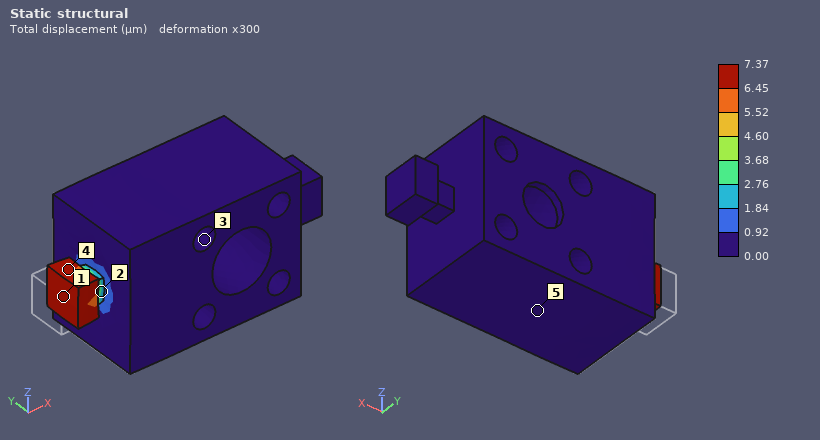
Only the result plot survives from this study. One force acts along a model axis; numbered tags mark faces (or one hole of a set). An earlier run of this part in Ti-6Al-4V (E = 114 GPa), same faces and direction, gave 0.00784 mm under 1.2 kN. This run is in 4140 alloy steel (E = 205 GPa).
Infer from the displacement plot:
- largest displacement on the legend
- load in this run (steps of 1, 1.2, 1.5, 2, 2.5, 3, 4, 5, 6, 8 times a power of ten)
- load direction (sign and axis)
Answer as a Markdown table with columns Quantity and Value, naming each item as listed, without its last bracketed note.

| Quantity | Value |
|---|---|
| largest displacement on the legend | 7.37 µm |
| load in this run | 2 kN |
| load direction | +X |
